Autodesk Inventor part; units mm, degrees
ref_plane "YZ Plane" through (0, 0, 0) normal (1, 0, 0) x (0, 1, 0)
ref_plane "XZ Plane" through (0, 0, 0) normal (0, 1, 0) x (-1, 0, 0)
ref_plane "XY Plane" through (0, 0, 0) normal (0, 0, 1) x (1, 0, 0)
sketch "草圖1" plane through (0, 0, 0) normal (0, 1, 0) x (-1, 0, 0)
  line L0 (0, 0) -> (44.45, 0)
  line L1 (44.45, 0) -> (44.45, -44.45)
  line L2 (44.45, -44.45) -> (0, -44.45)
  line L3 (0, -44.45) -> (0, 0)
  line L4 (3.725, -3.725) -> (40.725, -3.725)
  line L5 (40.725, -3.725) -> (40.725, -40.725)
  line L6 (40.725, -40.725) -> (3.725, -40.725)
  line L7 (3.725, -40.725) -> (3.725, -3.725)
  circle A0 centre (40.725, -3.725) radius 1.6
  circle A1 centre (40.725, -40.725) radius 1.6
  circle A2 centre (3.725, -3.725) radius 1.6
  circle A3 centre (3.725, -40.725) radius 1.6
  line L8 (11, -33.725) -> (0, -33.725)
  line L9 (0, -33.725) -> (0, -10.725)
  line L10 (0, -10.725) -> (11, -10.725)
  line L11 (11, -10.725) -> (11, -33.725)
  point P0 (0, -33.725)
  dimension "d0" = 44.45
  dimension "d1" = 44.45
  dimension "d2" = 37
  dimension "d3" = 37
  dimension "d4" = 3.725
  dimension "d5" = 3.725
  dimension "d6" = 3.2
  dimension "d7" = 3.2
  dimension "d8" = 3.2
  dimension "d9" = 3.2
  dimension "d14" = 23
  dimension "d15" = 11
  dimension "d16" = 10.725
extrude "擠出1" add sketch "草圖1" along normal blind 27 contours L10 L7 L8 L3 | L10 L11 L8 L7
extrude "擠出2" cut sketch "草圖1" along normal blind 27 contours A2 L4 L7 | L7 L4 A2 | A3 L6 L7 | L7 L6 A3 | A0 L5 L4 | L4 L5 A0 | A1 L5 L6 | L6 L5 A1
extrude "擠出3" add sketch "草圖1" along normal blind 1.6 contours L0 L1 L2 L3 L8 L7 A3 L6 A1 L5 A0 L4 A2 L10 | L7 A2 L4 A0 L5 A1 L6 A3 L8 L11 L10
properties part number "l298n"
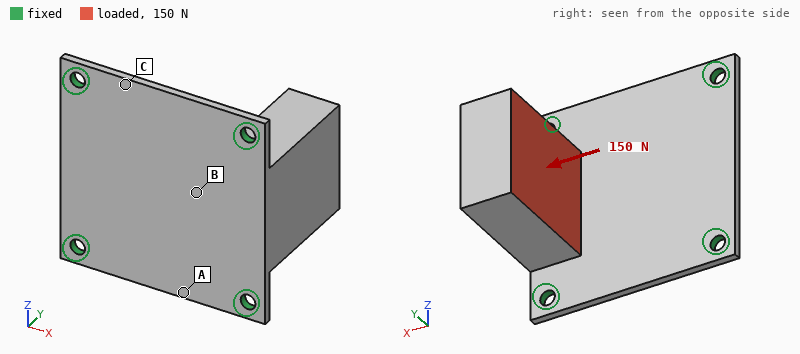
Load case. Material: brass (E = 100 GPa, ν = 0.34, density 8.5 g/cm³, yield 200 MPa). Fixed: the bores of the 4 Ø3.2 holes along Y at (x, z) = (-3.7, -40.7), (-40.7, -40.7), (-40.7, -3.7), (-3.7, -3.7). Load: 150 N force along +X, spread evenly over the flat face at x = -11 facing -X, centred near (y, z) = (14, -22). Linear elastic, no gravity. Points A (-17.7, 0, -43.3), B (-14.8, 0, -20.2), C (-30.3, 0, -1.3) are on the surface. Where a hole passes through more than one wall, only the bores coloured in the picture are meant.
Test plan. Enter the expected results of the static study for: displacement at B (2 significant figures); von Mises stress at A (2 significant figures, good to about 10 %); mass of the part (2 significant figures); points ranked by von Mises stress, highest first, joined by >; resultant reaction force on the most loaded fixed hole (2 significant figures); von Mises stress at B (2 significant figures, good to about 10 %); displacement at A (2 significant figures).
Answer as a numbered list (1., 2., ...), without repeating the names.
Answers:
1. 0.032 mm
2. 22 MPa
3. 81 g
4. B > A > C
5. 61 N
6. 36 MPa
7. 0.016 mm
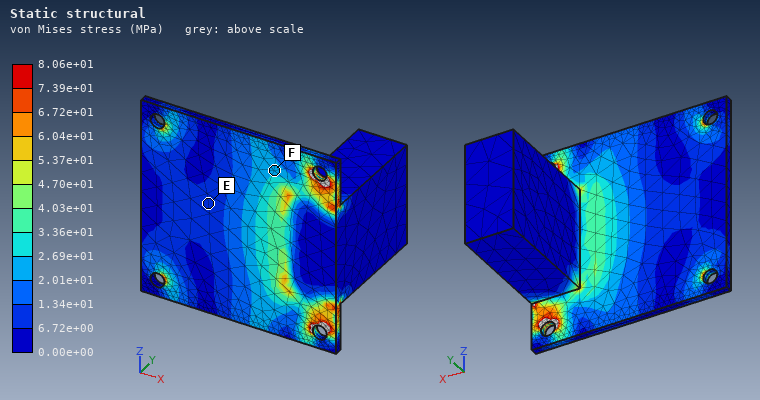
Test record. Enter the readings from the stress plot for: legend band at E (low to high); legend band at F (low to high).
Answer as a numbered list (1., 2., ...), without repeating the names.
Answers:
1. 6.72e+00 to 1.34e+01 MPa
2. 2.01e+01 to 2.69e+01 MPa
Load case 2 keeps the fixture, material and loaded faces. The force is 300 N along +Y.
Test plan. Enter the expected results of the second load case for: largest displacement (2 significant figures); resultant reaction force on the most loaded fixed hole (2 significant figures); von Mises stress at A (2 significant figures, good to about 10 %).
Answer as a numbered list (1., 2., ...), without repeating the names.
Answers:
1. 94 µm
2. 140 N
3. 24 MPa
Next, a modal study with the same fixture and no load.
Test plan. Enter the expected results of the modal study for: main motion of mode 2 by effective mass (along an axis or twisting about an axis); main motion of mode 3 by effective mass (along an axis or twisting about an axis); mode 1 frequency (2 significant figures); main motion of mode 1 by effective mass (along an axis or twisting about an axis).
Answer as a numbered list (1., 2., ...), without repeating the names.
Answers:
1. along Z
2. along Y
3. 960 Hz
4. along X
